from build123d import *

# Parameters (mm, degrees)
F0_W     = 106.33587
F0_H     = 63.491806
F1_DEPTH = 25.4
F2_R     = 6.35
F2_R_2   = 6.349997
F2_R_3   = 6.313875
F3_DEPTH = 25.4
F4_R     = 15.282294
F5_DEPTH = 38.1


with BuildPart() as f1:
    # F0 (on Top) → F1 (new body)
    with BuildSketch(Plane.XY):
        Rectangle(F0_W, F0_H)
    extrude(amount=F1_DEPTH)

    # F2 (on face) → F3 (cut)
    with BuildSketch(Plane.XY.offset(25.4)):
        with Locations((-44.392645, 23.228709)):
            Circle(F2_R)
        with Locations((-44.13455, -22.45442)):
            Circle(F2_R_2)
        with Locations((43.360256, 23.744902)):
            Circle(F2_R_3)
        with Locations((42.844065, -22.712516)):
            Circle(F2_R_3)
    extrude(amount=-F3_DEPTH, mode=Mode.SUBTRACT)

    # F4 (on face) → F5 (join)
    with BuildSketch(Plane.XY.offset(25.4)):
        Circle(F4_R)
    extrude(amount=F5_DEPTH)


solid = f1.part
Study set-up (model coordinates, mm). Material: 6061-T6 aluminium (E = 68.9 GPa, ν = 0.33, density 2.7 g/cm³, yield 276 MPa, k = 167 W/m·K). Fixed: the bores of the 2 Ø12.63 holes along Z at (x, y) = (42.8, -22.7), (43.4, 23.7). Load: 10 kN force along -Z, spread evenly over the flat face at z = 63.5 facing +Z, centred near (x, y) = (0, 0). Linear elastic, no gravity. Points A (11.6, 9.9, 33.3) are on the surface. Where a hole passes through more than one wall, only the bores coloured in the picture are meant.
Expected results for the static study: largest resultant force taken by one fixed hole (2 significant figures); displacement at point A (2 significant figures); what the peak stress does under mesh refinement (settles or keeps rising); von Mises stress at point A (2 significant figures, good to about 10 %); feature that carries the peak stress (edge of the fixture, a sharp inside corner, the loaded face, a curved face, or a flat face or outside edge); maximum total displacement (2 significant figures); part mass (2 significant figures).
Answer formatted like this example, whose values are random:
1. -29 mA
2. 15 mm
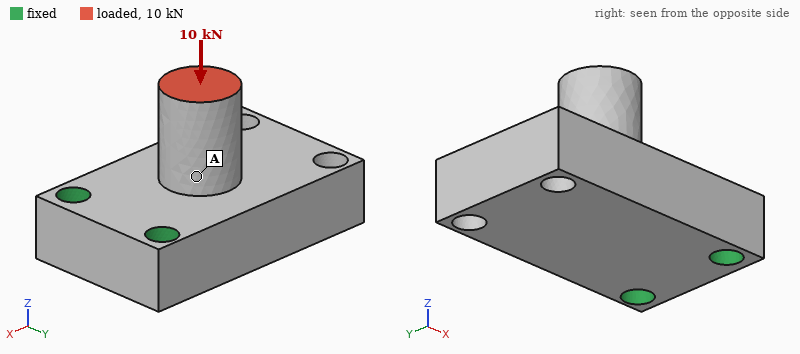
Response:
1. 5.2 kN
2. 0.050 mm
3. keeps rising
4. 14 MPa
5. edge of the fixture
6. 0.14 mm
7. 500 g
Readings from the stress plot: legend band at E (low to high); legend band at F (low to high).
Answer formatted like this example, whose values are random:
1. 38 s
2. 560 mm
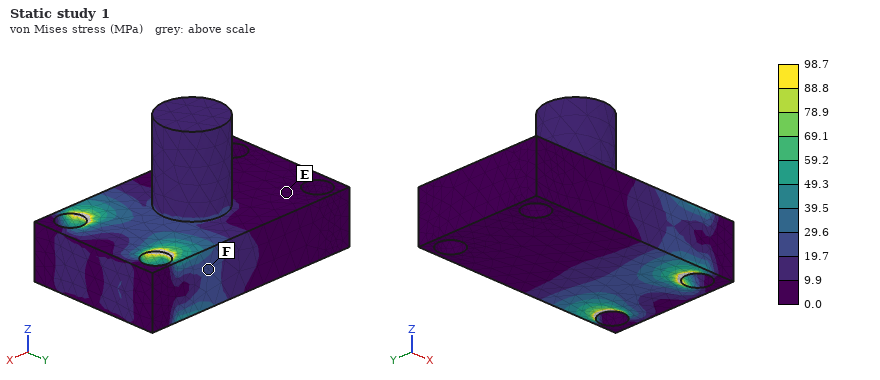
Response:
1. 0.0 to 9.9 MPa
2. 19.7 to 29.6 MPa
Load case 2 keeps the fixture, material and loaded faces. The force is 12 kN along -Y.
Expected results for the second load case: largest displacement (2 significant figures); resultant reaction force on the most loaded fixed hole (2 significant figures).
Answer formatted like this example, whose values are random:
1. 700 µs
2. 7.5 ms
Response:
1. 0.28 mm
2. 16 kN
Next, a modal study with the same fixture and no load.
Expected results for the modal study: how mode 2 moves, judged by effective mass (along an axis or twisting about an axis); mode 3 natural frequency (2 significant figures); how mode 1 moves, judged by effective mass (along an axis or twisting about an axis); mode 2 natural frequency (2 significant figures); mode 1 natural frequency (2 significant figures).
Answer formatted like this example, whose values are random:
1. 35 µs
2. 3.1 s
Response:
1. along Y
2. 5400 Hz
3. along Z
4. 4600 Hz
5. 2100 Hz
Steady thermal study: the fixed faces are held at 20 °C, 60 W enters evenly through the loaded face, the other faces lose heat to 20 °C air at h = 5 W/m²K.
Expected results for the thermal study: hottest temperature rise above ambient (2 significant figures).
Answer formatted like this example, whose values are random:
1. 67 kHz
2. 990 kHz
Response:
1. 30 K
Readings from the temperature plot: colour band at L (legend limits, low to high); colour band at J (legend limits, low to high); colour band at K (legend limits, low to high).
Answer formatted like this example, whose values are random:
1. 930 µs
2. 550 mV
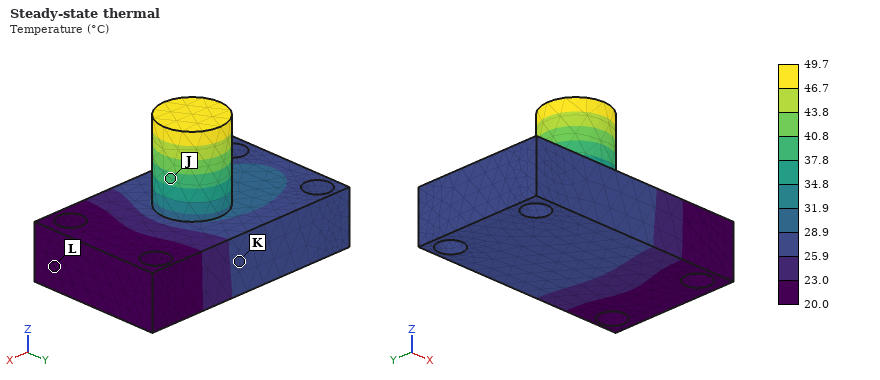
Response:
1. 20.0 to 23.0 °C
2. 37.8 to 40.8 °C
3. 25.9 to 28.9 °C
